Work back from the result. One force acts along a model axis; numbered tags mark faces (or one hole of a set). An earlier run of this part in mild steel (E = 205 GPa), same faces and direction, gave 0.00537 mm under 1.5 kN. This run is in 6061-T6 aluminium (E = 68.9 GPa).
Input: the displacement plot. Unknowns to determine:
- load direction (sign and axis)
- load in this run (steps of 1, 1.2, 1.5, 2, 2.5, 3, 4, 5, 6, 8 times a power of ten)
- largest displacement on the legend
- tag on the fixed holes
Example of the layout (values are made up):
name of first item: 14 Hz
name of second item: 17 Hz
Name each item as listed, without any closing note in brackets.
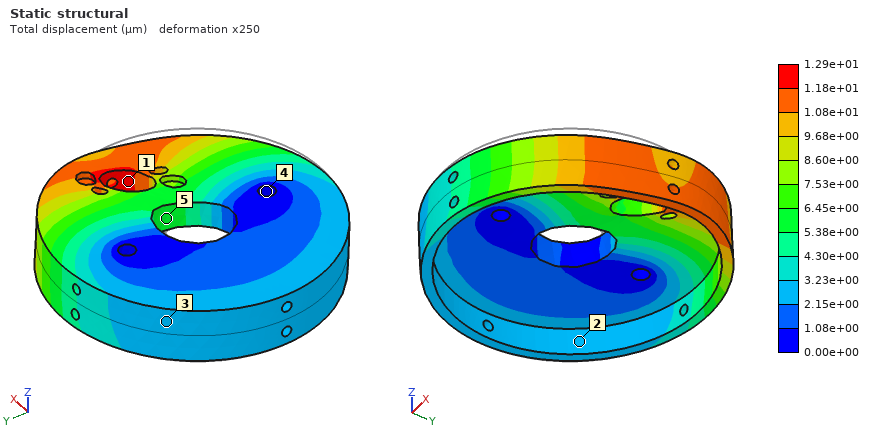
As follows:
load direction: +Y
load in this run: 1.2 kN
largest displacement on the legend: 1.29e+01 µm
tag on the fixed holes: 4
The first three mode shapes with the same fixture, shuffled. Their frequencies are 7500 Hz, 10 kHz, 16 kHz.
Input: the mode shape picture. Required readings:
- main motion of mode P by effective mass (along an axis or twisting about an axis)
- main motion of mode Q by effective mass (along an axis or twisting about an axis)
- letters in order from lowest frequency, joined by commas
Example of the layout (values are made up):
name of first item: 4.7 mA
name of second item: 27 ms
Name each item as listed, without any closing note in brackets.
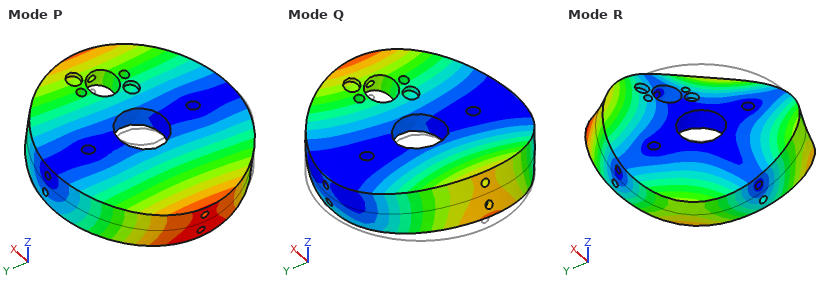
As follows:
main motion of mode P by effective mass: twisting about Y
main motion of mode Q by effective mass: along Z
letters in order from lowest frequency, joined by commas: P, Q, R
